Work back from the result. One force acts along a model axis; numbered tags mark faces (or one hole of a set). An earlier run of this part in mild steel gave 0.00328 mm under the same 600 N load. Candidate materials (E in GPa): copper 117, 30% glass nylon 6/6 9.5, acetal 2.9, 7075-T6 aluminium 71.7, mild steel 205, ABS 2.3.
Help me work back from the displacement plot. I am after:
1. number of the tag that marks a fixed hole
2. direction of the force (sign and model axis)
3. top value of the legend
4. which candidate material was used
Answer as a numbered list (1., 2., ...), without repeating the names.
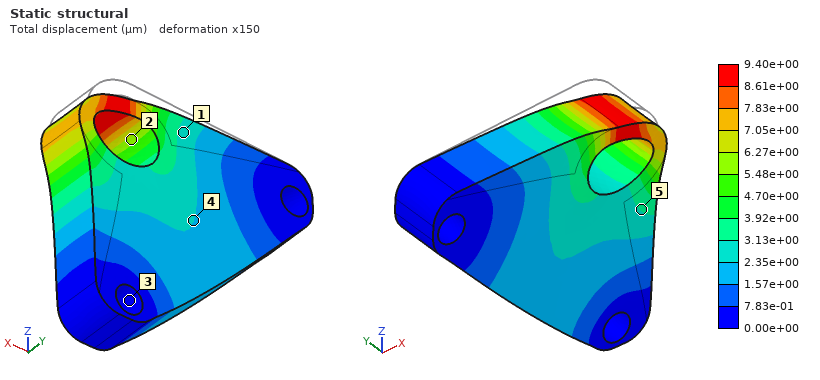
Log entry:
1. 3
2. -Z
3. 9.40e+00 µm
4. 7075-T6 aluminium
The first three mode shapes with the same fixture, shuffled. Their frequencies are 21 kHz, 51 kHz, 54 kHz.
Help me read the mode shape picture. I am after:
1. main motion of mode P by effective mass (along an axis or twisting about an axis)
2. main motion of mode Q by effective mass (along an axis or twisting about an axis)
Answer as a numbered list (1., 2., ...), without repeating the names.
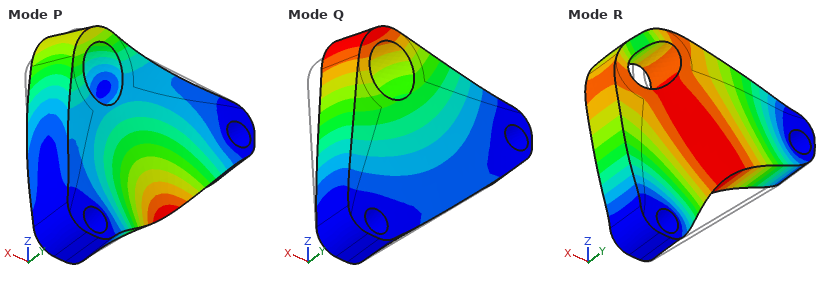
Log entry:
1. along Y
2. along Y
